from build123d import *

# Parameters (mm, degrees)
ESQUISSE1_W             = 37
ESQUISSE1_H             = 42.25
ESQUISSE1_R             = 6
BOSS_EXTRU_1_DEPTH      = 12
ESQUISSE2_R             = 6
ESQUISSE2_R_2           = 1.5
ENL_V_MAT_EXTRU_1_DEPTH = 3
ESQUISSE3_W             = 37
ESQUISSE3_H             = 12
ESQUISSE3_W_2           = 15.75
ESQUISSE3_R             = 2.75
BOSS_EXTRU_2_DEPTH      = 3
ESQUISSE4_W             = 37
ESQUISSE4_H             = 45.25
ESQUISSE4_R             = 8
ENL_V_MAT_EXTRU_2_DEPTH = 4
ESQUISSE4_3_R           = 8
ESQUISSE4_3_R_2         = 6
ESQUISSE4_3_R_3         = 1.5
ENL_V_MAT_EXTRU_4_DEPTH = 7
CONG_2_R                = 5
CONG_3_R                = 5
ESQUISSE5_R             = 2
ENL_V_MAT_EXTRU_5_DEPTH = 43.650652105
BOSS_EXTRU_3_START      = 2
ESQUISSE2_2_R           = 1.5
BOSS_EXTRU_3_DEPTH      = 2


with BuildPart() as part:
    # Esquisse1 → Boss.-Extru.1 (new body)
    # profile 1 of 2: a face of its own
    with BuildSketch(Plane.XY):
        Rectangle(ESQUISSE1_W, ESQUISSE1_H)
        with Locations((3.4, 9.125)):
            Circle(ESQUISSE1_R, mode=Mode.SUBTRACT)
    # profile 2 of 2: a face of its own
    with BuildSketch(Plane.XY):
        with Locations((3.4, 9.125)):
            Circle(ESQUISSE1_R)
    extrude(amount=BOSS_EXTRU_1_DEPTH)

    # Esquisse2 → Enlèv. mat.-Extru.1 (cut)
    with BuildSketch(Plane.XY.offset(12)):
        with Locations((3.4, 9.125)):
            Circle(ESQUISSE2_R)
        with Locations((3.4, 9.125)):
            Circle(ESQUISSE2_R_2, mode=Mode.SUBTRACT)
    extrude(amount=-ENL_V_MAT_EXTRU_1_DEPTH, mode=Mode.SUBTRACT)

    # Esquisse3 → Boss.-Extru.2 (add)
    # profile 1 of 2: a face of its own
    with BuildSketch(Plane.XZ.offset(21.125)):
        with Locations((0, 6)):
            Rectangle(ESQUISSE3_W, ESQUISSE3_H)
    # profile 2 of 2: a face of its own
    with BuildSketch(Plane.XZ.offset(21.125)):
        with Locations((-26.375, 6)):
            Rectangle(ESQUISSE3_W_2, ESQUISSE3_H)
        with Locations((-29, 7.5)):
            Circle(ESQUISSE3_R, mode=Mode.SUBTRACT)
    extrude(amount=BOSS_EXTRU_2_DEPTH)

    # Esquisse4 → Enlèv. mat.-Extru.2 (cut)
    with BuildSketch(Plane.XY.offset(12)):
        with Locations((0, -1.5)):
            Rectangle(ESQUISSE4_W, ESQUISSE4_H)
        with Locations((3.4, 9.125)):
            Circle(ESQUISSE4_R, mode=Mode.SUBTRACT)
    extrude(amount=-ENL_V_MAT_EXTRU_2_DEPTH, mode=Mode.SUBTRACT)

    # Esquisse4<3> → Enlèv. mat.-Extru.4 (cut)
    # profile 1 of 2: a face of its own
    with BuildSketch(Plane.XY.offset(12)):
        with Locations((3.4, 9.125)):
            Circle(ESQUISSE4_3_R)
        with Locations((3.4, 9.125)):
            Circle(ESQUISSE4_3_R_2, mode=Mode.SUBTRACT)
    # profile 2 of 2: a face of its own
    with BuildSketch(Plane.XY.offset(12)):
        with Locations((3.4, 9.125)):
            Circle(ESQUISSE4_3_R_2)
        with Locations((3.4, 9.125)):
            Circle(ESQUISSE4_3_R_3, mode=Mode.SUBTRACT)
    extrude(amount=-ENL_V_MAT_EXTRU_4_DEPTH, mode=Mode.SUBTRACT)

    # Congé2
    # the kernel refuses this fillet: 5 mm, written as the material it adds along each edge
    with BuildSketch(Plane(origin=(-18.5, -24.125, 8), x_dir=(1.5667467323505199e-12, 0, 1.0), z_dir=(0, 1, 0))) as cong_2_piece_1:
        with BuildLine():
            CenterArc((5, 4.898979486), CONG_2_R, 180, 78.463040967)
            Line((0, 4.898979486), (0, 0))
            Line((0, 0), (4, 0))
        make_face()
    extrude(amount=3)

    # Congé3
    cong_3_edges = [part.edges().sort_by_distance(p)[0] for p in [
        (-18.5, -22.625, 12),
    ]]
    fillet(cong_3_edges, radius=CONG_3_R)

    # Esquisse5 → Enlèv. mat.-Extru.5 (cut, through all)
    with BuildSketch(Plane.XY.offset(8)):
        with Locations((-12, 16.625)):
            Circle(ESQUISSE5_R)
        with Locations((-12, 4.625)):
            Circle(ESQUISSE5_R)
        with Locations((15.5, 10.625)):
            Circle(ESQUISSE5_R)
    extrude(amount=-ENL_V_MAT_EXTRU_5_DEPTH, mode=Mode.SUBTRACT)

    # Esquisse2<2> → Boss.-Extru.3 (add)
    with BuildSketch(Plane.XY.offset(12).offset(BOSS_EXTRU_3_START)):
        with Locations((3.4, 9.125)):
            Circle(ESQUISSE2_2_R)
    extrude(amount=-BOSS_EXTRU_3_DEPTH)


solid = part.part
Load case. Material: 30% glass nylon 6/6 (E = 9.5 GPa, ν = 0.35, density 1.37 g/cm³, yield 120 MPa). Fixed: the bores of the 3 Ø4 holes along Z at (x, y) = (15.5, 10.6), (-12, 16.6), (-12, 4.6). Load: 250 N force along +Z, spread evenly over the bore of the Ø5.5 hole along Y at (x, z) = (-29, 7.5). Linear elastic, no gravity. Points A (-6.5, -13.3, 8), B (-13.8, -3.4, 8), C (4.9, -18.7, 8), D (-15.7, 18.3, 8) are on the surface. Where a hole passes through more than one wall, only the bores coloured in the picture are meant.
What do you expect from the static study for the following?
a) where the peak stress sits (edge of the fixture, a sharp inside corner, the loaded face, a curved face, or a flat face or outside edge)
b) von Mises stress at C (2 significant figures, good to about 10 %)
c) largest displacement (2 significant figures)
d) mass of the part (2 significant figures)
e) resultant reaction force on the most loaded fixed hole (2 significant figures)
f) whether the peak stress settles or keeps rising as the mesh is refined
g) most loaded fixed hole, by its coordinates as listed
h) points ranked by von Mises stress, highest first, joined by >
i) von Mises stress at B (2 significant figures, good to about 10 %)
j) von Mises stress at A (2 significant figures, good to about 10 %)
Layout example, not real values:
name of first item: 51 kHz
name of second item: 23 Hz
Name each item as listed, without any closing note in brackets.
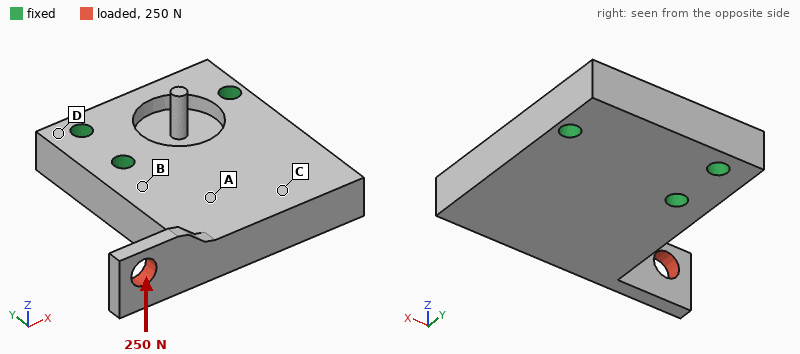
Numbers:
where the peak stress sits: edge of the fixture
von Mises stress at C: 10 MPa
largest displacement: 0.77 mm
mass of the part: 18 g
resultant reaction force on the most loaded fixed hole: 490 N
whether the peak stress settles or keeps rising as the mesh is refined: keeps rising
most loaded fixed hole, by its coordinates as listed: (-12, 4.6)
points ranked by von Mises stress, highest first, joined by >: B > A > C > D
von Mises stress at B: 27 MPa
von Mises stress at A: 21 MPa
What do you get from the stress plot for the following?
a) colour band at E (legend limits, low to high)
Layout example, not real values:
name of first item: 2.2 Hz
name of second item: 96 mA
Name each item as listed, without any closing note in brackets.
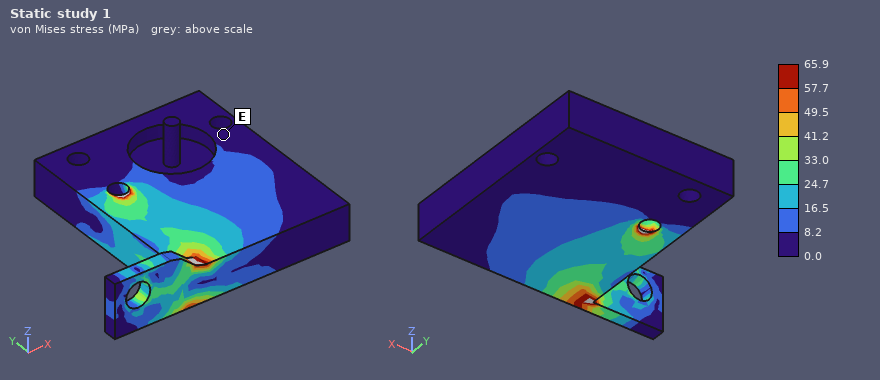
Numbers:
colour band at E: 0.0 to 8.2 MPa
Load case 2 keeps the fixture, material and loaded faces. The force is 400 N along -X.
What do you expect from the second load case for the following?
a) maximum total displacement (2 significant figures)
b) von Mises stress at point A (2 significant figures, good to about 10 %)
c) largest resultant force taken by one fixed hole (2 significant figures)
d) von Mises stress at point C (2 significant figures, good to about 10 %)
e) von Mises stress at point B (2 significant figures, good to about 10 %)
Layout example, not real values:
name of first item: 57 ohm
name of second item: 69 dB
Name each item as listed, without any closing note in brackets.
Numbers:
maximum total displacement: 0.23 mm
von Mises stress at point A: 8.4 MPa
largest resultant force taken by one fixed hole: 450 N
von Mises stress at point C: 4.7 MPa
von Mises stress at point B: 5.3 MPa
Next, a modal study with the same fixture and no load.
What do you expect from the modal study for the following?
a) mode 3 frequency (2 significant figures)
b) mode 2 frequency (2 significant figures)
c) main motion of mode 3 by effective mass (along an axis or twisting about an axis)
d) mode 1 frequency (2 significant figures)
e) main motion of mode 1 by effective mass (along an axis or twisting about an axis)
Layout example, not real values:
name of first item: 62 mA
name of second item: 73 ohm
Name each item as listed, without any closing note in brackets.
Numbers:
mode 3 frequency: 4200 Hz
mode 2 frequency: 4000 Hz
main motion of mode 3 by effective mass: twisting about Y
mode 1 frequency: 2800 Hz
main motion of mode 1 by effective mass: along Z
